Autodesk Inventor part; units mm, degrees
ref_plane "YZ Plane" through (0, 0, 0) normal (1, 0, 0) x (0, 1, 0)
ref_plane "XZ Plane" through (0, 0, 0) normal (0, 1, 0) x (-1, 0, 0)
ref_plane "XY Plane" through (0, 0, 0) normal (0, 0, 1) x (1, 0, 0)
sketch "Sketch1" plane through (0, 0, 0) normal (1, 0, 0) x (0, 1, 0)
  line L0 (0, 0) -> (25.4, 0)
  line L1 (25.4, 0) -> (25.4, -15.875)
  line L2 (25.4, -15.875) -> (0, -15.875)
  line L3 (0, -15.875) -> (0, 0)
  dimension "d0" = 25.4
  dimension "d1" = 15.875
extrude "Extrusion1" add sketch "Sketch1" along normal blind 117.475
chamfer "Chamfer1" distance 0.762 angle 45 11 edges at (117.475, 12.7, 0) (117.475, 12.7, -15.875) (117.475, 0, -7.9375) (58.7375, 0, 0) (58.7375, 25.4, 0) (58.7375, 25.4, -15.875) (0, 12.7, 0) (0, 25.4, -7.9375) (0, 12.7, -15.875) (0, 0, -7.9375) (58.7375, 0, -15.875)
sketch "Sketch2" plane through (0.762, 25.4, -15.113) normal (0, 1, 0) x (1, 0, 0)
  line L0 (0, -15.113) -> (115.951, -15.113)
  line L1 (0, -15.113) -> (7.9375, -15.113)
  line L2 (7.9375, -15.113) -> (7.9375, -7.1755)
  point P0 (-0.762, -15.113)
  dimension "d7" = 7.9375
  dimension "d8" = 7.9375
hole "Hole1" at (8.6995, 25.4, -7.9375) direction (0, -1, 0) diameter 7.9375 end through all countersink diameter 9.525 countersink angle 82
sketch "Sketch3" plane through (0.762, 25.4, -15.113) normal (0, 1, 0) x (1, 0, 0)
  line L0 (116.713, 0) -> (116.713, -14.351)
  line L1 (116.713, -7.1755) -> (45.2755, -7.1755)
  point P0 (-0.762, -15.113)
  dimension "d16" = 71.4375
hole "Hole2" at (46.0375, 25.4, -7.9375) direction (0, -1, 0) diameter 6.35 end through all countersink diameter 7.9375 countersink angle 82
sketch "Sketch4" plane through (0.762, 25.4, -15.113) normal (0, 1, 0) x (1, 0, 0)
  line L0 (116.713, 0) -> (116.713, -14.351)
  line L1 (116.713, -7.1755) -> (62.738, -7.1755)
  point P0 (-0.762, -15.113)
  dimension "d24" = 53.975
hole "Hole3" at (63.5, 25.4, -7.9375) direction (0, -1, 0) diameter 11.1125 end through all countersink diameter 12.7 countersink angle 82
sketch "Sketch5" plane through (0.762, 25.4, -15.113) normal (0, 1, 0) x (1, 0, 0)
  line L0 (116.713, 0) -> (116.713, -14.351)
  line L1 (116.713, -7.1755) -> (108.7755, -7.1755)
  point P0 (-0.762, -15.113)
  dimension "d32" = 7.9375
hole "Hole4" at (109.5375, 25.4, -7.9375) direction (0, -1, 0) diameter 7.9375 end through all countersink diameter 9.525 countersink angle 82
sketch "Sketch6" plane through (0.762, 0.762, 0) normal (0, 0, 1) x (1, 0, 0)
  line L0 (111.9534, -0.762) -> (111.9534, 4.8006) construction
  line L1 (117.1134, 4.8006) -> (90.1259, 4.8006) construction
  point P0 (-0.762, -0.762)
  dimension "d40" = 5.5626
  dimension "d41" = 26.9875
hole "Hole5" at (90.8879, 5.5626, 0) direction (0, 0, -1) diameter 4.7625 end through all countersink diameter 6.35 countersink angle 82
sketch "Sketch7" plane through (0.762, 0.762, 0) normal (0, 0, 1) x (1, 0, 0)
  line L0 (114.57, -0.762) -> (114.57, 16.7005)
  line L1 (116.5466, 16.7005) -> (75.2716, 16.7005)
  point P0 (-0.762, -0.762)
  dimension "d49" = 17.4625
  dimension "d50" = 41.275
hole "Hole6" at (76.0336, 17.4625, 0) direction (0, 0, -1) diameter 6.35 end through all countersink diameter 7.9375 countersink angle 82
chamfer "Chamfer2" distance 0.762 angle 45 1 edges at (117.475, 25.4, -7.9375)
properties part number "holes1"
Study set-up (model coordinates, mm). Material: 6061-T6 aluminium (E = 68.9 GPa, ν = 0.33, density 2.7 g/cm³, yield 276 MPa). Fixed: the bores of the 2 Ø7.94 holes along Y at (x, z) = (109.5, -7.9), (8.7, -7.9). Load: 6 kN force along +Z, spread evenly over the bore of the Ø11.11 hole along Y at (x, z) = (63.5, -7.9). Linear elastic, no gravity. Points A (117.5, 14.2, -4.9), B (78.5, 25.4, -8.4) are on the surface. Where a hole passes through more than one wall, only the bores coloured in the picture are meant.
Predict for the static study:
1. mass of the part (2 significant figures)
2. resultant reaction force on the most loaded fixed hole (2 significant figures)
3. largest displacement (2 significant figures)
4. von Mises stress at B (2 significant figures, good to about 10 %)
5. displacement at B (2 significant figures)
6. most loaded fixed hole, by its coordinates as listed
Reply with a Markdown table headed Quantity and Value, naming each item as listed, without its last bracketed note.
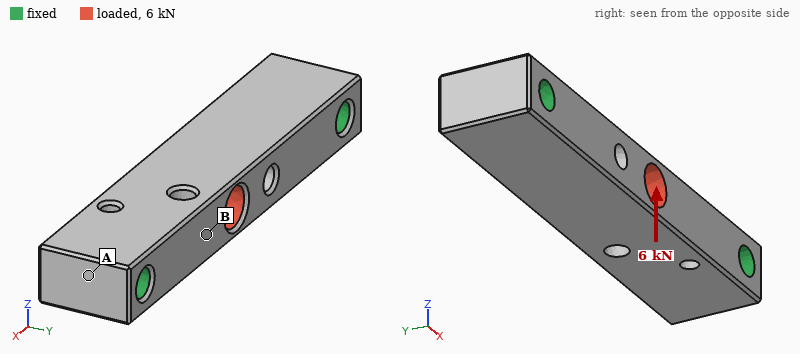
| Quantity | Value |
|---|---|
| mass of the part | 110 g |
| resultant reaction force on the most loaded fixed hole | 3.4 kN |
| largest displacement | 84 µm |
| von Mises stress at B | 37 MPa |
| displacement at B | 55 µm |
| most loaded fixed hole, by its coordinates as listed | (109.5, -7.9) |
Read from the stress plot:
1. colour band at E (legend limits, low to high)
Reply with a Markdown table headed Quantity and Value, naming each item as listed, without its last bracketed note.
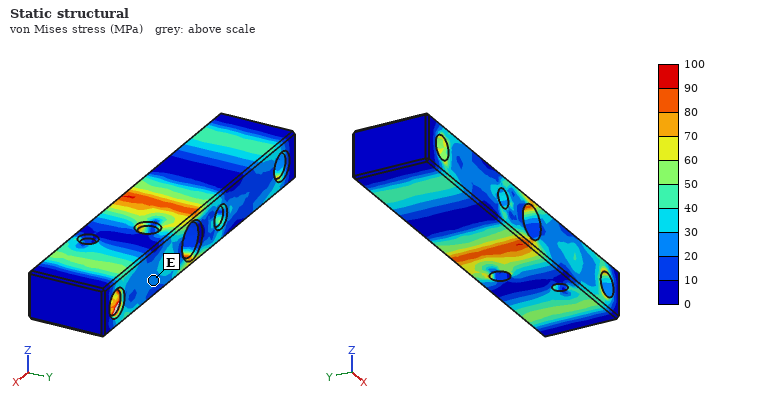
| Quantity | Value |
|---|---|
| colour band at E | 20 to 30 MPa |
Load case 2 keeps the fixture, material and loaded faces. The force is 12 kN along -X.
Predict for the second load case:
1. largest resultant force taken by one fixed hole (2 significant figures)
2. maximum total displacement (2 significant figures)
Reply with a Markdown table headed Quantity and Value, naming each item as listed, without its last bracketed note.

| Quantity | Value |
|---|---|
| largest resultant force taken by one fixed hole | 6.3 kN |
| maximum total displacement | 12 µm |
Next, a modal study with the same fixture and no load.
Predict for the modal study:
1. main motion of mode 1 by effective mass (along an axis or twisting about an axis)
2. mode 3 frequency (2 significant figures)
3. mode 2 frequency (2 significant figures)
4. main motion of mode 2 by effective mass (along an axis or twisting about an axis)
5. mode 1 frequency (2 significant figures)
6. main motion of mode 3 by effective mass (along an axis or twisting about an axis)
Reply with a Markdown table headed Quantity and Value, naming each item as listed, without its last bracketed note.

| Quantity | Value |
|---|---|
| main motion of mode 1 by effective mass | along Z |
| mode 3 frequency | 14 kHz |
| mode 2 frequency | 10 kHz |
| main motion of mode 2 by effective mass | along Y |
| mode 1 frequency | 7400 Hz |
| main motion of mode 3 by effective mass | twisting about X |
